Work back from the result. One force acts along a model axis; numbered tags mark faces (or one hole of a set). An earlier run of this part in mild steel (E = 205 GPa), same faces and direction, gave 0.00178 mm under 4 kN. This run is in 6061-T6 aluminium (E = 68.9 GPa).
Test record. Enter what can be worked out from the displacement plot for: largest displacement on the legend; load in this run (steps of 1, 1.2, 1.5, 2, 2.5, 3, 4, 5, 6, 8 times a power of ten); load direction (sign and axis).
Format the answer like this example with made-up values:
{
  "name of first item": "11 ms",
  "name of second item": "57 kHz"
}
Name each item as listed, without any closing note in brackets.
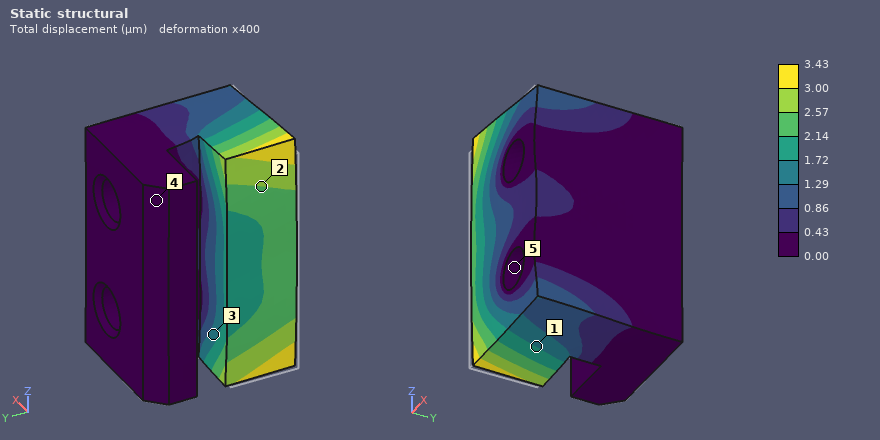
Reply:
{
  "largest displacement on the legend": "3.43 µm",
  "load in this run": "2.5 kN",
  "load direction": "+X"
}
